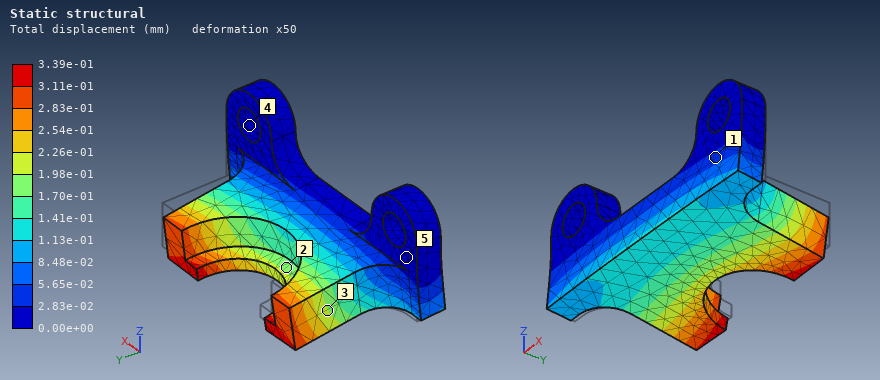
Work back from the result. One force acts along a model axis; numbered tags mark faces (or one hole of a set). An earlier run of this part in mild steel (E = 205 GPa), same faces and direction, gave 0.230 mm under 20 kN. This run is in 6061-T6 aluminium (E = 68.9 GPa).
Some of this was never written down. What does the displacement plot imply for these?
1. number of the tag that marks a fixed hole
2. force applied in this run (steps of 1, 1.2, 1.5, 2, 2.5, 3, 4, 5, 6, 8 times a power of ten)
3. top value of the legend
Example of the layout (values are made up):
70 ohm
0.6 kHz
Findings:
4
10 kN
3.39e-01 mm
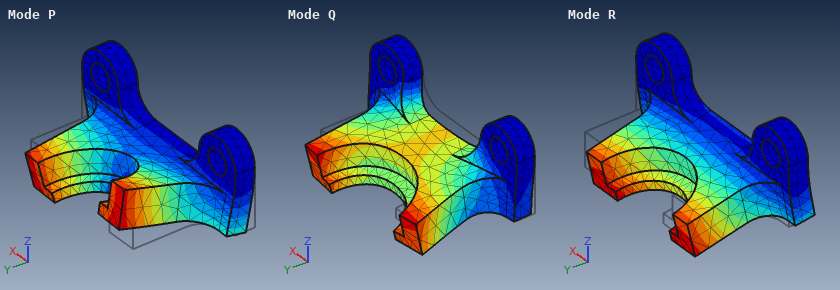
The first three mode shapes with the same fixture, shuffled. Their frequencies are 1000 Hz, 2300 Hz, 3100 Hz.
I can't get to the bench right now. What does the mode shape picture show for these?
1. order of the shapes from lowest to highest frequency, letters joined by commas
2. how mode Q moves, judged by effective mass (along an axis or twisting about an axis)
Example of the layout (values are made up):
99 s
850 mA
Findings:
R, P, Q
along Y
